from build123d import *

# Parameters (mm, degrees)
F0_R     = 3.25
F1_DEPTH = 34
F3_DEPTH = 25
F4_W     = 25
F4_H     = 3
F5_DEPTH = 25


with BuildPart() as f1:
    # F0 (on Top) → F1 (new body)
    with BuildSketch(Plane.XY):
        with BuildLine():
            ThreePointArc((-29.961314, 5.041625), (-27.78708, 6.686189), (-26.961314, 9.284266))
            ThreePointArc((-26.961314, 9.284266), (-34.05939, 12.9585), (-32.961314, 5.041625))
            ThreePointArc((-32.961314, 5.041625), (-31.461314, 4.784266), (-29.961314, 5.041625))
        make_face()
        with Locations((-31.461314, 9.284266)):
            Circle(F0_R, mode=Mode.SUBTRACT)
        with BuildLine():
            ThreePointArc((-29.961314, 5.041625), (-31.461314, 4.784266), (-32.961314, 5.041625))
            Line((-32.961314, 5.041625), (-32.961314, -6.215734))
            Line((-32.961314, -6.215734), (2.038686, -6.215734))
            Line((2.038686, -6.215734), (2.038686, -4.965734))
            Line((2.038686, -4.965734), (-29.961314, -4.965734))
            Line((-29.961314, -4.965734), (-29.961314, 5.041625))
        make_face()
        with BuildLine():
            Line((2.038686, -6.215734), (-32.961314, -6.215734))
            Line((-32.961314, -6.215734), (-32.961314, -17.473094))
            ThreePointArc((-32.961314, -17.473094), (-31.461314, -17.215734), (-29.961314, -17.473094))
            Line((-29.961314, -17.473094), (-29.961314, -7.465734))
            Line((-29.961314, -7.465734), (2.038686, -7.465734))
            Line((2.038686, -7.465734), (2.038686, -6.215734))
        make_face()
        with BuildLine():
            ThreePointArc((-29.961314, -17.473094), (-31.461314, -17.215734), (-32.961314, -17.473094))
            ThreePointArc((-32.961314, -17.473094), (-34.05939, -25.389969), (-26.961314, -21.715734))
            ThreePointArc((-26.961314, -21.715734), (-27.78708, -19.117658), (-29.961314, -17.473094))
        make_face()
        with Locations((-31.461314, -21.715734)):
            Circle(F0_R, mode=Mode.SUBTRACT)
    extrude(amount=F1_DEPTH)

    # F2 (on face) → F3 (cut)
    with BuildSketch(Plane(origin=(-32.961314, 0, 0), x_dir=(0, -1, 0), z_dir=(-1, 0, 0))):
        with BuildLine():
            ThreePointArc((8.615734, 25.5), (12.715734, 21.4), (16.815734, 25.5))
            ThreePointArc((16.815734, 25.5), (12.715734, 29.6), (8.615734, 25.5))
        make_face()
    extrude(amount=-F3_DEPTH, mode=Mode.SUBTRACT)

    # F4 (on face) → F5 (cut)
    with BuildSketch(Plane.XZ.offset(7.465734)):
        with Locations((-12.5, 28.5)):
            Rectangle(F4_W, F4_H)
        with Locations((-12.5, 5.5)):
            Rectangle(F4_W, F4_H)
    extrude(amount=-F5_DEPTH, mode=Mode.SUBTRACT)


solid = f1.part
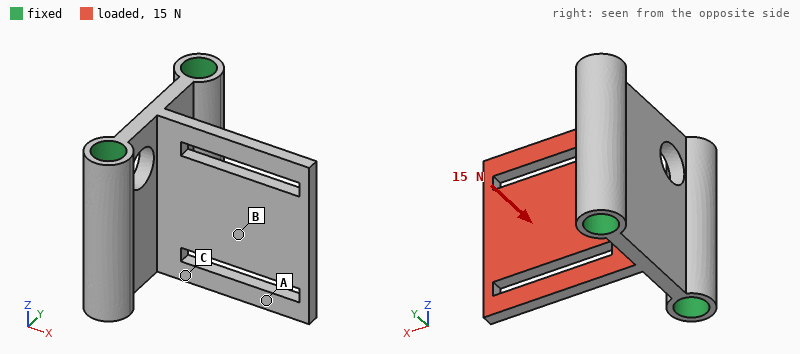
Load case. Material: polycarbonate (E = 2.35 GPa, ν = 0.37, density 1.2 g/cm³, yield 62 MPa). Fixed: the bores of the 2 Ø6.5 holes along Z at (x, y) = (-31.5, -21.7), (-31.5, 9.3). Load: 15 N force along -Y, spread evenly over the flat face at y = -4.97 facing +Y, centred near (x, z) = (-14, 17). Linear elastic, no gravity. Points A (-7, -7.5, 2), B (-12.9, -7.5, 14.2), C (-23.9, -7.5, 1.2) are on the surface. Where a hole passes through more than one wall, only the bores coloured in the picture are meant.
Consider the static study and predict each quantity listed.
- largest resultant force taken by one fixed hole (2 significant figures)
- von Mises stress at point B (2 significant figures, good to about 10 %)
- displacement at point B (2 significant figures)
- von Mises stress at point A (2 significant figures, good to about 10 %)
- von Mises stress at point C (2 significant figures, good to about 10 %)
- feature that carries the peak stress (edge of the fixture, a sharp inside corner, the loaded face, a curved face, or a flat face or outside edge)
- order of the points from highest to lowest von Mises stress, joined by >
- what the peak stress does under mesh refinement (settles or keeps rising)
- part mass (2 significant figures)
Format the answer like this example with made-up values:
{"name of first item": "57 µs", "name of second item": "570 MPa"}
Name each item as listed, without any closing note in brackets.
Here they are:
{"largest resultant force taken by one fixed hole": "18 N", "von Mises stress at point B": "1.7 MPa", "displacement at point B": "0.31 mm", "von Mises stress at point A": "0.72 MPa", "von Mises stress at point C": "5.3 MPa", "feature that carries the peak stress": "a sharp inside corner", "order of the points from highest to lowest von Mises stress, joined by >": "C > B > A", "what the peak stress does under mesh refinement": "keeps rising", "part mass": "7.8 g"}
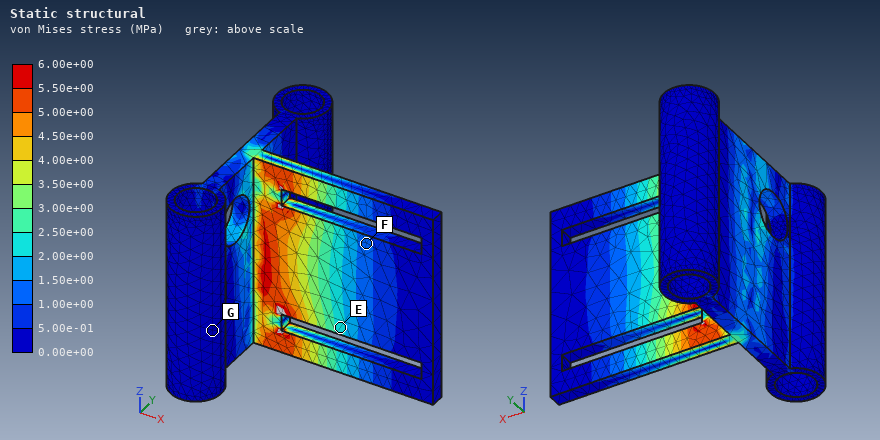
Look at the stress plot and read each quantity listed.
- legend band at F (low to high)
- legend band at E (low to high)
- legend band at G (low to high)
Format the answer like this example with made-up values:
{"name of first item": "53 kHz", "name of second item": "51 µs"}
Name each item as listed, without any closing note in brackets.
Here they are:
{"legend band at F": "1.00e+00 to 1.50e+00 MPa", "legend band at E": "2.00e+00 to 2.50e+00 MPa", "legend band at G": "0.00e+00 to 5.00e-01 MPa"}
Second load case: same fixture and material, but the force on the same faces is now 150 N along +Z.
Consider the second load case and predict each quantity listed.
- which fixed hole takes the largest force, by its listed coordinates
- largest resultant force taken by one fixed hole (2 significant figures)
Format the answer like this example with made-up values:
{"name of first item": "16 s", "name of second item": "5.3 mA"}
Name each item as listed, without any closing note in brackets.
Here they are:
{"which fixed hole takes the largest force, by its listed coordinates": "(-31.5, 9.3)", "largest resultant force taken by one fixed hole": "89 N"}
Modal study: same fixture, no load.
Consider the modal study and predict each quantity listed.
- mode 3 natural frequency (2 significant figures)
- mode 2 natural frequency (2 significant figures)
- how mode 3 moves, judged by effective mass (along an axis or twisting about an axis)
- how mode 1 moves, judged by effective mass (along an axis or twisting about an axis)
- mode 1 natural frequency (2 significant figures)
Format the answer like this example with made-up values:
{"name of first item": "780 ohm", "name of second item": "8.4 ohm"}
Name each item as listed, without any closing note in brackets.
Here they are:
{"mode 3 natural frequency": "1800 Hz", "mode 2 natural frequency": "1200 Hz", "how mode 3 moves, judged by effective mass": "along Z", "how mode 1 moves, judged by effective mass": "along Y", "mode 1 natural frequency": "530 Hz"}
